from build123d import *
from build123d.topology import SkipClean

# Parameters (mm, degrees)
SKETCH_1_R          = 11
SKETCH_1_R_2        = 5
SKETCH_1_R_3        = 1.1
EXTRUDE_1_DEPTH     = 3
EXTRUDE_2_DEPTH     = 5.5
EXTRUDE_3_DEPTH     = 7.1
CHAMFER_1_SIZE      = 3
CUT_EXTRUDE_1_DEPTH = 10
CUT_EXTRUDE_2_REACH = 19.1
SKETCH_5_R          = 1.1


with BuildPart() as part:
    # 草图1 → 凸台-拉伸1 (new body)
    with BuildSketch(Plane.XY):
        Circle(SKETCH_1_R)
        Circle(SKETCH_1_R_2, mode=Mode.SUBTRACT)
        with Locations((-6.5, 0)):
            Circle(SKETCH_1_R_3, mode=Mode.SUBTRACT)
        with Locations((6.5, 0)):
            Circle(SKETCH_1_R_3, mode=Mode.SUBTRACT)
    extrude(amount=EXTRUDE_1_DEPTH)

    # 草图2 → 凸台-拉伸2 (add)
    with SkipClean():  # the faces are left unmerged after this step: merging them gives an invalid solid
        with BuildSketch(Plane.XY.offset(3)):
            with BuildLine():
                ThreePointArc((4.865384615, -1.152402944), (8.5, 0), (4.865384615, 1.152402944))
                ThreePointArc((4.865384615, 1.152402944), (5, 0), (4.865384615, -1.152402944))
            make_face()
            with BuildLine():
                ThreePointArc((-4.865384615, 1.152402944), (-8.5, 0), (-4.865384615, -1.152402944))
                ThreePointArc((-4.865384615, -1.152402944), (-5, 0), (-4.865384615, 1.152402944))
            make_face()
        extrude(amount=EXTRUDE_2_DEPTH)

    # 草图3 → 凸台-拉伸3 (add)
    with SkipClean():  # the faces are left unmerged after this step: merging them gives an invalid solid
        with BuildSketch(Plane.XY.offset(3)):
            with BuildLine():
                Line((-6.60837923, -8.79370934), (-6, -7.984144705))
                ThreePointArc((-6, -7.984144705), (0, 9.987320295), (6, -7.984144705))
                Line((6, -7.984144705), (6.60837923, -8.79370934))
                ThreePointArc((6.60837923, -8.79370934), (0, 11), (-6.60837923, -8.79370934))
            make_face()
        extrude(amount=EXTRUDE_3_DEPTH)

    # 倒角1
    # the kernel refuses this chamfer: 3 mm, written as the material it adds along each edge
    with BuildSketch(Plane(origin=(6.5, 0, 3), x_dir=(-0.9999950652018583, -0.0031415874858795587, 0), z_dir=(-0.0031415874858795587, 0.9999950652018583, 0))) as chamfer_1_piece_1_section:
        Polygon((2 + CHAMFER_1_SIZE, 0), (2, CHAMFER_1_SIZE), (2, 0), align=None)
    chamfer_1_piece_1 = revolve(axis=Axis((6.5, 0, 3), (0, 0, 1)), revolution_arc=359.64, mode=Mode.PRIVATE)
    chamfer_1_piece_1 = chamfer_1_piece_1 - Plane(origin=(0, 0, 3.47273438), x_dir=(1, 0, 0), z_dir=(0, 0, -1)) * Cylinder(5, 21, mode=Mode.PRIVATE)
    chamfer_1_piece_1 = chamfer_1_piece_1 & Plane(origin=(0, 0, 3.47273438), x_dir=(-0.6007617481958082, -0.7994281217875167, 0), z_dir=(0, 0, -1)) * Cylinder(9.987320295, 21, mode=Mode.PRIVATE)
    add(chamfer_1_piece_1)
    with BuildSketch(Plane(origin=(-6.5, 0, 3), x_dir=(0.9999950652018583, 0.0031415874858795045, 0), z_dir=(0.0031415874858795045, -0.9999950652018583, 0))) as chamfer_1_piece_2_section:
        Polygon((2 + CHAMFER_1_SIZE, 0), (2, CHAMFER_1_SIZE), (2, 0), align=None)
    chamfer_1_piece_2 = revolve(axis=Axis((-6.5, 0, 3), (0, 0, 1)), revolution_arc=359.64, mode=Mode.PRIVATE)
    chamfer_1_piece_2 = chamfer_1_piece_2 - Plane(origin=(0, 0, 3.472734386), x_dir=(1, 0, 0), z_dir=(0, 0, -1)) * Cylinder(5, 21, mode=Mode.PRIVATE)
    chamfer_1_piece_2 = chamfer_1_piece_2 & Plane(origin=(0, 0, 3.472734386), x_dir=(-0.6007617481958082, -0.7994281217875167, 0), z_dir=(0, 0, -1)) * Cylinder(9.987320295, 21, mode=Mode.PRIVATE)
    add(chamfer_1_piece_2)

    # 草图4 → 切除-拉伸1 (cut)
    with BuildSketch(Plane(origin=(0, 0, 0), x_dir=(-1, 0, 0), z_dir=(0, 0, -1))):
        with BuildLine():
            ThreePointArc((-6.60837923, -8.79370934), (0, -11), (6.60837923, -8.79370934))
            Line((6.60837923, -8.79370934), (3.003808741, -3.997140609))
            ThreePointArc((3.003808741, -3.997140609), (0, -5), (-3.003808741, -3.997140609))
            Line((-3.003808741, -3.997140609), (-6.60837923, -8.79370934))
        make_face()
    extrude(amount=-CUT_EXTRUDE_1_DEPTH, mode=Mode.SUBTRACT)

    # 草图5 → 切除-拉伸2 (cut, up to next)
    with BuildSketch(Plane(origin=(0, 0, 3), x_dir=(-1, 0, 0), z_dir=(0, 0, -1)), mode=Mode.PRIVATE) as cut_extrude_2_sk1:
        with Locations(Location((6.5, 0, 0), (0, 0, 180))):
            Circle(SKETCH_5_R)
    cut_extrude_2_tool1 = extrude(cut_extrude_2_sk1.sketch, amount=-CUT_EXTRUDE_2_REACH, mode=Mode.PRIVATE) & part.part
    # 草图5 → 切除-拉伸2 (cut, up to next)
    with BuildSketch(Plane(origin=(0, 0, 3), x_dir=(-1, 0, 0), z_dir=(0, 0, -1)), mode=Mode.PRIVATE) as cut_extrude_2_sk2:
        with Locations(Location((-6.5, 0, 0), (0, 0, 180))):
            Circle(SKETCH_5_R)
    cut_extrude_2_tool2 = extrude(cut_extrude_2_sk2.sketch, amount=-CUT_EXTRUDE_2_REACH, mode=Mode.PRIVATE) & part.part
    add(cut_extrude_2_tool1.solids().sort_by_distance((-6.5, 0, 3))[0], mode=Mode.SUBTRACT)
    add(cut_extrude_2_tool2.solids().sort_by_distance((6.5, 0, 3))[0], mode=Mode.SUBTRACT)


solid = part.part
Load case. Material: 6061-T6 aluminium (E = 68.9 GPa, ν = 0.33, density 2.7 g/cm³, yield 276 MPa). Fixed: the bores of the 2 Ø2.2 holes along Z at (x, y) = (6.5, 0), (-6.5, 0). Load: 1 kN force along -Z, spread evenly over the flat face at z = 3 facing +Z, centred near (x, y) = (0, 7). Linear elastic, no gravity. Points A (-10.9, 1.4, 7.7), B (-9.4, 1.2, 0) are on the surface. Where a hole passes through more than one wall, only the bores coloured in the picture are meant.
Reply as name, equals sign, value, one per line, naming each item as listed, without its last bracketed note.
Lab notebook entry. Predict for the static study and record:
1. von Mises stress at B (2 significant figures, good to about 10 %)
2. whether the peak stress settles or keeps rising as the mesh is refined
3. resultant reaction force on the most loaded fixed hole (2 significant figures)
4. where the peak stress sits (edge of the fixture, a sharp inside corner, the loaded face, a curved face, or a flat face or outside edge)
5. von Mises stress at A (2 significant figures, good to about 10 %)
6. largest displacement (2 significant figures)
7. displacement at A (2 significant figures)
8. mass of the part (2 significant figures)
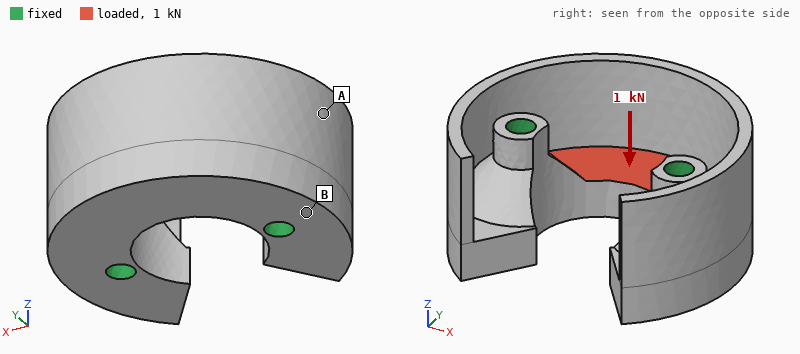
von Mises stress at B = 45 MPa
whether the peak stress settles or keeps rising as the mesh is refined = keeps rising
resultant reaction force on the most loaded fixed hole = 500 N
where the peak stress sits = edge of the fixture
von Mises stress at A = 20 MPa
largest displacement = 57 µm
displacement at A = 15 µm
mass of the part = 3.4 g
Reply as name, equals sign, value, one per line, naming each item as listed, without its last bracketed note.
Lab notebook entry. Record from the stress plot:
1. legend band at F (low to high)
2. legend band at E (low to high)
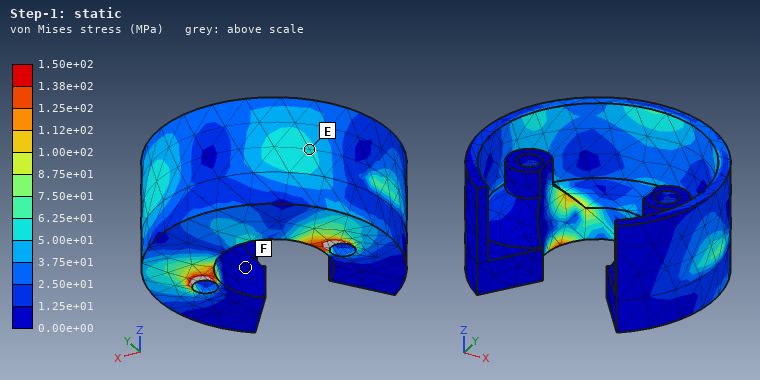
legend band at F = 0.00e+00 to 1.25e+01 MPa
legend band at E = 5.00e+01 to 6.25e+01 MPa
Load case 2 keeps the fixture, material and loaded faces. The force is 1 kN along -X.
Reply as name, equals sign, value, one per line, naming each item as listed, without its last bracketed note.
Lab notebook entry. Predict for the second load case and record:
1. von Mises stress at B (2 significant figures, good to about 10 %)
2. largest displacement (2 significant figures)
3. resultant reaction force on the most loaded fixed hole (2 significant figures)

von Mises stress at B = 26 MPa
largest displacement = 17 µm
resultant reaction force on the most loaded fixed hole = 570 N
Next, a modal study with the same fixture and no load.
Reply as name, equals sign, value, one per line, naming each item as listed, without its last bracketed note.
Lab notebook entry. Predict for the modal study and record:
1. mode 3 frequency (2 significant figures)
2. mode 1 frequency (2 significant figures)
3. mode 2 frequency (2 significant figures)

mode 3 frequency = 23 kHz
mode 1 frequency = 21 kHz
mode 2 frequency = 22 kHz
